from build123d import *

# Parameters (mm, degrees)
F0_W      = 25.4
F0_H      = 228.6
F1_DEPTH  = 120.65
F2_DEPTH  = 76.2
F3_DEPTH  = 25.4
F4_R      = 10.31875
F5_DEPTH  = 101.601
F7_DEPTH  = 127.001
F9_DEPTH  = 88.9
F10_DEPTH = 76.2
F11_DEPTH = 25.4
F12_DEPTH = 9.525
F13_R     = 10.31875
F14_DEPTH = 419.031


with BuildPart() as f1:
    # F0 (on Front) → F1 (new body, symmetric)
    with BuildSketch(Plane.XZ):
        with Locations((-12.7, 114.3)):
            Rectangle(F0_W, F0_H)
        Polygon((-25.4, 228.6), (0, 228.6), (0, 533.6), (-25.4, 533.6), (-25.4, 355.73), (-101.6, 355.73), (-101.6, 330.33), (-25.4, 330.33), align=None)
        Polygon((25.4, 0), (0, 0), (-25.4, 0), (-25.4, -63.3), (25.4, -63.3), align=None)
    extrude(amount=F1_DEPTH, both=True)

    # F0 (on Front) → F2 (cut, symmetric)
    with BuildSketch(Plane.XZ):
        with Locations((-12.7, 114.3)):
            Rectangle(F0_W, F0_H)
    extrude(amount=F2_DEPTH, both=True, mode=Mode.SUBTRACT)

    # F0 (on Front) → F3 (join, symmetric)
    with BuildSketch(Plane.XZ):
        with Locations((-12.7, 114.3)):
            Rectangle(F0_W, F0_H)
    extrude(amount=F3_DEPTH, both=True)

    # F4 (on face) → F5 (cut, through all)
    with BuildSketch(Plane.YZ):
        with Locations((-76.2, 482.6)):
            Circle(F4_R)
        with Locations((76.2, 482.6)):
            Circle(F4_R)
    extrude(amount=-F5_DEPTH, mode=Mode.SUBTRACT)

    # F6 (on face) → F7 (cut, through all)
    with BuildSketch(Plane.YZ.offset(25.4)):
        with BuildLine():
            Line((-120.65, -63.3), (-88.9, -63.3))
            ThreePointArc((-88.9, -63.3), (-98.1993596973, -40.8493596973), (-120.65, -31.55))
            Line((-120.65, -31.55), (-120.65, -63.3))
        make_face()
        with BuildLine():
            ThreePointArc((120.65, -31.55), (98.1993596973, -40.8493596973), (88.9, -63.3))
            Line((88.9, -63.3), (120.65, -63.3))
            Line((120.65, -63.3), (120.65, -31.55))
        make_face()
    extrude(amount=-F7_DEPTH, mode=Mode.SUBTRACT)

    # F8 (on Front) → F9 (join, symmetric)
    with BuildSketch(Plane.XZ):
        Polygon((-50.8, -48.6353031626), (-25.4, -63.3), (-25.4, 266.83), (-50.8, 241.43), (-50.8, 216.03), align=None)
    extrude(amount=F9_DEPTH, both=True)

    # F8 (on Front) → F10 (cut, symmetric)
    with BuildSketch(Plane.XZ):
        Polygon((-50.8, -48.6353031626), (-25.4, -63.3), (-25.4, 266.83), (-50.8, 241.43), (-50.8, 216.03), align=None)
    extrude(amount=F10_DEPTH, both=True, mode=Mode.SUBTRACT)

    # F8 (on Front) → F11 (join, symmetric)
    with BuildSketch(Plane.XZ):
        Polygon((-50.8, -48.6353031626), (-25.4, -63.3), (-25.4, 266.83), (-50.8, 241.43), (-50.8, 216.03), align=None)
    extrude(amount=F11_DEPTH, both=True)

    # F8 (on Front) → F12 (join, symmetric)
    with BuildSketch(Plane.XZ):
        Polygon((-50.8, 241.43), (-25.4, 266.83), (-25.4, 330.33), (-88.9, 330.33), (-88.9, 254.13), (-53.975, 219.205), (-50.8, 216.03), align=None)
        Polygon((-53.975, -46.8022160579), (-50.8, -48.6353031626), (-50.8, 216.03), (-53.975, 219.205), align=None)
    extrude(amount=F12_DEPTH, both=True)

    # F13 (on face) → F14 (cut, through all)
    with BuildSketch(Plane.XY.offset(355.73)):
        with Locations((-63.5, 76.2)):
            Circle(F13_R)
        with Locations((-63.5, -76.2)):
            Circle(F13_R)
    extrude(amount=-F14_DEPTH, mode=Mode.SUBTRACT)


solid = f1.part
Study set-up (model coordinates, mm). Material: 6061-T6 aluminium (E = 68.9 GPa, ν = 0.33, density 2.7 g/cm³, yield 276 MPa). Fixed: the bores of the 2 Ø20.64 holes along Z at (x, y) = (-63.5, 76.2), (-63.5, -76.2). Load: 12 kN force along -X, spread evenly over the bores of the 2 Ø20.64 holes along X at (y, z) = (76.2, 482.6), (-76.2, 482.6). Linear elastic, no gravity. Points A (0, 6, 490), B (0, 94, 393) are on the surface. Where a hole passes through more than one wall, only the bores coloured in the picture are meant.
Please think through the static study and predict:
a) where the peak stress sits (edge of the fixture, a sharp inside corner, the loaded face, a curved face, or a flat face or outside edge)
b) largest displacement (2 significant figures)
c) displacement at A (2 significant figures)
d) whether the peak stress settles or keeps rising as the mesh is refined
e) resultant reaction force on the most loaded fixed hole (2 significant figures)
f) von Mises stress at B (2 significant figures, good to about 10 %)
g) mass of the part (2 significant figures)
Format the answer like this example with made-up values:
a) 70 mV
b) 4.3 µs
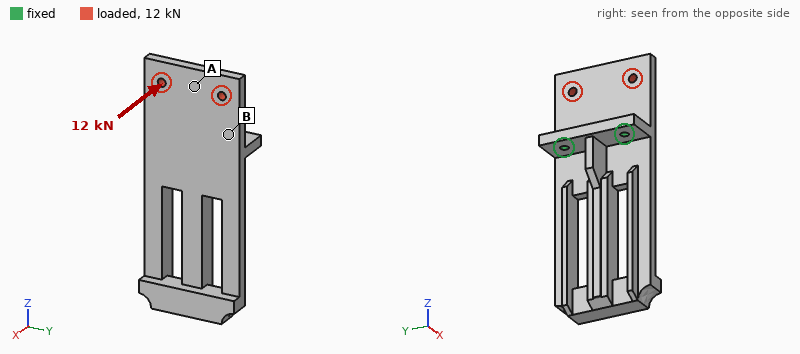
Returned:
a) edge of the fixture
b) 1.2 mm
c) 0.90 mm
d) keeps rising
e) 6.6 kN
f) 39 MPa
g) 12 kg
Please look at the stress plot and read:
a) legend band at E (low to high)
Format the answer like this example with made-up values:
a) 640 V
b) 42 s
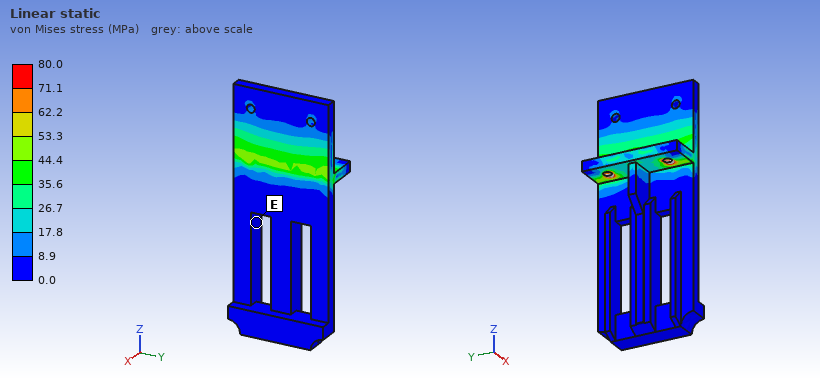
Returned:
a) 0.0 to 8.9 MPa
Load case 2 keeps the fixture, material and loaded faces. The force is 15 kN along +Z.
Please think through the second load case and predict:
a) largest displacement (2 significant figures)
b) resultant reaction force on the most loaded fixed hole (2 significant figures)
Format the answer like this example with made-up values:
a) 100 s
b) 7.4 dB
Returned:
a) 0.31 mm
b) 7.5 kN
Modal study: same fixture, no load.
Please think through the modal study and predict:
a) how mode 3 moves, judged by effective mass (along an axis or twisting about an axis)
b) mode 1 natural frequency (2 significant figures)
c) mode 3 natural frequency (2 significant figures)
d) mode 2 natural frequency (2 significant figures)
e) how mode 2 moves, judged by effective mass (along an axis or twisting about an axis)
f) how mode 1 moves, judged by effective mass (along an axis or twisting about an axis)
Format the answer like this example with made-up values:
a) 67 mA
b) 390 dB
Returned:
a) twisting about Z
b) 140 Hz
c) 440 Hz
d) 330 Hz
e) along Y
f) along X
